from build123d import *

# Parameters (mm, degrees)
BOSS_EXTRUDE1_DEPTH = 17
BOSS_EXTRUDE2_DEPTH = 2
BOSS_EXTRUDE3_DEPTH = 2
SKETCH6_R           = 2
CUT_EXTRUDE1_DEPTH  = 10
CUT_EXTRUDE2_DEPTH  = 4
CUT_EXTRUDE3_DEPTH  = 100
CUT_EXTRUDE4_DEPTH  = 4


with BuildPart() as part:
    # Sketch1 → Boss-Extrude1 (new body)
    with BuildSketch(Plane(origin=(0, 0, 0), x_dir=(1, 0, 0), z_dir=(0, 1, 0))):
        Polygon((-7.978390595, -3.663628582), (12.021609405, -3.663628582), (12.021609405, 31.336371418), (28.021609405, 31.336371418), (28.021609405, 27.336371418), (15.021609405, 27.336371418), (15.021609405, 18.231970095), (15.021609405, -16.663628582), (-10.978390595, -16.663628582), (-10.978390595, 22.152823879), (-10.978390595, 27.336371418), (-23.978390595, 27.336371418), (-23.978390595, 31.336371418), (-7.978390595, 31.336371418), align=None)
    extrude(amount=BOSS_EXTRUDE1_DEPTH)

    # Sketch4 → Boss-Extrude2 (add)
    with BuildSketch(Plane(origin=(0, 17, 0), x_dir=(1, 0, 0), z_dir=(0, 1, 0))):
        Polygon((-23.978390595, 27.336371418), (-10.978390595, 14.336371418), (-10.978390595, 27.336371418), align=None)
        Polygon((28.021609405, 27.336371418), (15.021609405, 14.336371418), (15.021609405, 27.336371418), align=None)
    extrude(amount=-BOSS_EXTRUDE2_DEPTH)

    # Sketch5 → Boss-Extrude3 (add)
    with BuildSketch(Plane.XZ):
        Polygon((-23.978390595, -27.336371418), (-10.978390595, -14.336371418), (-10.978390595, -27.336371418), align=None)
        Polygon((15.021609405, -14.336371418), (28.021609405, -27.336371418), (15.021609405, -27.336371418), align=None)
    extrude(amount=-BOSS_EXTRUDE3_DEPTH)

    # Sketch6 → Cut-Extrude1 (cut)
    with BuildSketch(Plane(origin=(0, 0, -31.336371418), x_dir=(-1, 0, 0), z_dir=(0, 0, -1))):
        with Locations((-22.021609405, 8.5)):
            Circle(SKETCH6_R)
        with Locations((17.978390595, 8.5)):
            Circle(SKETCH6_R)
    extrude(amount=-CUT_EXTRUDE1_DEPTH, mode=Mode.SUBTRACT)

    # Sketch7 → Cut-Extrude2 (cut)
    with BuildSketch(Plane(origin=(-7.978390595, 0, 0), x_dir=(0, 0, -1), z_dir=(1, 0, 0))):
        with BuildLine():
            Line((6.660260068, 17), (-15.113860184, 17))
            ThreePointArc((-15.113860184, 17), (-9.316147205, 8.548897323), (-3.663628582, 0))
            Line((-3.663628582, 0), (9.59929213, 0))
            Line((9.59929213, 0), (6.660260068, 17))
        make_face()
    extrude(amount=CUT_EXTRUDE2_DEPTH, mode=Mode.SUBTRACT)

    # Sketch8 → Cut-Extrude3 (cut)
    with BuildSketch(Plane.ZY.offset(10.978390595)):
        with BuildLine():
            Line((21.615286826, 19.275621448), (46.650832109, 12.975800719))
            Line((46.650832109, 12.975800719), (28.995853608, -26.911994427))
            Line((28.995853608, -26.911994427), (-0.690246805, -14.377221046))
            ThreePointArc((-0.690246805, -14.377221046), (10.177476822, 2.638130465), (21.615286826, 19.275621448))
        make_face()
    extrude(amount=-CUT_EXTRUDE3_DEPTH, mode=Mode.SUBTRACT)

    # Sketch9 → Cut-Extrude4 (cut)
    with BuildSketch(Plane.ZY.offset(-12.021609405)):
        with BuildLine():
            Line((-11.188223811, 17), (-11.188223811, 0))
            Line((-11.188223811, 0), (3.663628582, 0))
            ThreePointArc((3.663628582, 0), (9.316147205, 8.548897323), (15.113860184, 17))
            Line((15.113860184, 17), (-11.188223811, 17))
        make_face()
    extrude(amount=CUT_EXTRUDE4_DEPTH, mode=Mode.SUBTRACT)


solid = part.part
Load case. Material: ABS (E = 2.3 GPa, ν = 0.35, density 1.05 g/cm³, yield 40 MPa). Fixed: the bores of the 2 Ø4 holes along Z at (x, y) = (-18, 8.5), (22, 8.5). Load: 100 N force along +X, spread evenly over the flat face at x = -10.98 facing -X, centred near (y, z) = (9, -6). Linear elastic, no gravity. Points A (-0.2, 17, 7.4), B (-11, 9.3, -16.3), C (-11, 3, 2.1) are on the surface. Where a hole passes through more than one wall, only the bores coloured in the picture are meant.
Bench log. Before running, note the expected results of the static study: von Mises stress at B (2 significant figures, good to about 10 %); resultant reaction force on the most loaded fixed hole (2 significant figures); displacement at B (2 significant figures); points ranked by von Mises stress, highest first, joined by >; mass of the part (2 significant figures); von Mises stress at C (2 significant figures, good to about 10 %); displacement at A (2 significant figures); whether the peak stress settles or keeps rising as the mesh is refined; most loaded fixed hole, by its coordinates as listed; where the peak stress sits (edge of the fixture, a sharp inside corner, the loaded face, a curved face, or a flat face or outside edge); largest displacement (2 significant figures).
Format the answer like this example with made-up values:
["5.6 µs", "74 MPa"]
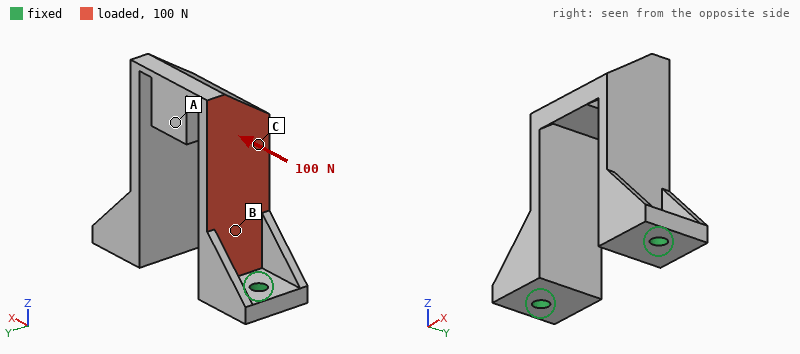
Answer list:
["5.5 MPa", "78 N", "0.25 mm", "C > B > A", "10 g", "9.2 MPa", "0.84 mm", "keeps rising", "(-18, 8.5)", "edge of the fixture", "0.86 mm"]
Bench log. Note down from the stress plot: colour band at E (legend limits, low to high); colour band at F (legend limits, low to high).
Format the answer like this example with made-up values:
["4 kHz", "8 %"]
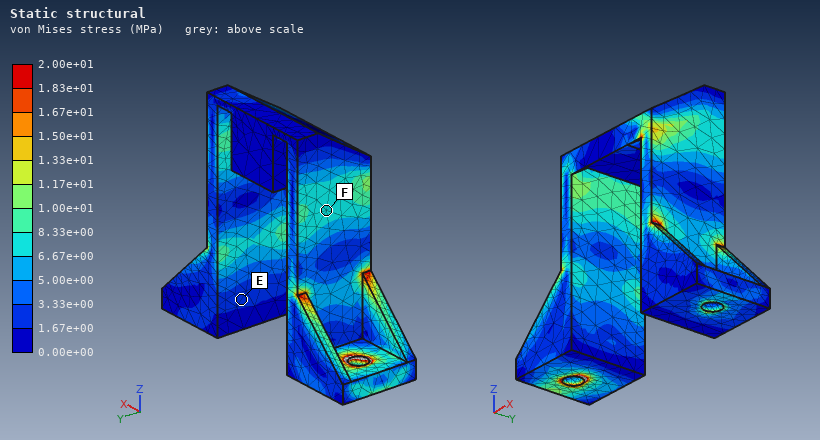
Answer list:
["1.67e+00 to 3.33e+00 MPa", "6.67e+00 to 8.33e+00 MPa"]
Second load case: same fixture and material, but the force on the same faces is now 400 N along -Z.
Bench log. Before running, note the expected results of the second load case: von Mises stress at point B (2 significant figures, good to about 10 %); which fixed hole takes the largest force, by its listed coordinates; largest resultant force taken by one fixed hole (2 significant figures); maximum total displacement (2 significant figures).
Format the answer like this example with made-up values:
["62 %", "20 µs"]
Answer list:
["14 MPa", "(-18, 8.5)", "400 N", "0.59 mm"]
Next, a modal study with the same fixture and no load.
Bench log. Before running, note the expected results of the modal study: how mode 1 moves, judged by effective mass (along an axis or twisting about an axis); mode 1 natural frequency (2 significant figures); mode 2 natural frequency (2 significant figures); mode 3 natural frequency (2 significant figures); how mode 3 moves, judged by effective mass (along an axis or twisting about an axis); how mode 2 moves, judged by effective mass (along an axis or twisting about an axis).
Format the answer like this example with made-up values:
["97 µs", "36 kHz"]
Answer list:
["along Y", "600 Hz", "620 Hz", "1200 Hz", "twisting about Z", "along X"]
